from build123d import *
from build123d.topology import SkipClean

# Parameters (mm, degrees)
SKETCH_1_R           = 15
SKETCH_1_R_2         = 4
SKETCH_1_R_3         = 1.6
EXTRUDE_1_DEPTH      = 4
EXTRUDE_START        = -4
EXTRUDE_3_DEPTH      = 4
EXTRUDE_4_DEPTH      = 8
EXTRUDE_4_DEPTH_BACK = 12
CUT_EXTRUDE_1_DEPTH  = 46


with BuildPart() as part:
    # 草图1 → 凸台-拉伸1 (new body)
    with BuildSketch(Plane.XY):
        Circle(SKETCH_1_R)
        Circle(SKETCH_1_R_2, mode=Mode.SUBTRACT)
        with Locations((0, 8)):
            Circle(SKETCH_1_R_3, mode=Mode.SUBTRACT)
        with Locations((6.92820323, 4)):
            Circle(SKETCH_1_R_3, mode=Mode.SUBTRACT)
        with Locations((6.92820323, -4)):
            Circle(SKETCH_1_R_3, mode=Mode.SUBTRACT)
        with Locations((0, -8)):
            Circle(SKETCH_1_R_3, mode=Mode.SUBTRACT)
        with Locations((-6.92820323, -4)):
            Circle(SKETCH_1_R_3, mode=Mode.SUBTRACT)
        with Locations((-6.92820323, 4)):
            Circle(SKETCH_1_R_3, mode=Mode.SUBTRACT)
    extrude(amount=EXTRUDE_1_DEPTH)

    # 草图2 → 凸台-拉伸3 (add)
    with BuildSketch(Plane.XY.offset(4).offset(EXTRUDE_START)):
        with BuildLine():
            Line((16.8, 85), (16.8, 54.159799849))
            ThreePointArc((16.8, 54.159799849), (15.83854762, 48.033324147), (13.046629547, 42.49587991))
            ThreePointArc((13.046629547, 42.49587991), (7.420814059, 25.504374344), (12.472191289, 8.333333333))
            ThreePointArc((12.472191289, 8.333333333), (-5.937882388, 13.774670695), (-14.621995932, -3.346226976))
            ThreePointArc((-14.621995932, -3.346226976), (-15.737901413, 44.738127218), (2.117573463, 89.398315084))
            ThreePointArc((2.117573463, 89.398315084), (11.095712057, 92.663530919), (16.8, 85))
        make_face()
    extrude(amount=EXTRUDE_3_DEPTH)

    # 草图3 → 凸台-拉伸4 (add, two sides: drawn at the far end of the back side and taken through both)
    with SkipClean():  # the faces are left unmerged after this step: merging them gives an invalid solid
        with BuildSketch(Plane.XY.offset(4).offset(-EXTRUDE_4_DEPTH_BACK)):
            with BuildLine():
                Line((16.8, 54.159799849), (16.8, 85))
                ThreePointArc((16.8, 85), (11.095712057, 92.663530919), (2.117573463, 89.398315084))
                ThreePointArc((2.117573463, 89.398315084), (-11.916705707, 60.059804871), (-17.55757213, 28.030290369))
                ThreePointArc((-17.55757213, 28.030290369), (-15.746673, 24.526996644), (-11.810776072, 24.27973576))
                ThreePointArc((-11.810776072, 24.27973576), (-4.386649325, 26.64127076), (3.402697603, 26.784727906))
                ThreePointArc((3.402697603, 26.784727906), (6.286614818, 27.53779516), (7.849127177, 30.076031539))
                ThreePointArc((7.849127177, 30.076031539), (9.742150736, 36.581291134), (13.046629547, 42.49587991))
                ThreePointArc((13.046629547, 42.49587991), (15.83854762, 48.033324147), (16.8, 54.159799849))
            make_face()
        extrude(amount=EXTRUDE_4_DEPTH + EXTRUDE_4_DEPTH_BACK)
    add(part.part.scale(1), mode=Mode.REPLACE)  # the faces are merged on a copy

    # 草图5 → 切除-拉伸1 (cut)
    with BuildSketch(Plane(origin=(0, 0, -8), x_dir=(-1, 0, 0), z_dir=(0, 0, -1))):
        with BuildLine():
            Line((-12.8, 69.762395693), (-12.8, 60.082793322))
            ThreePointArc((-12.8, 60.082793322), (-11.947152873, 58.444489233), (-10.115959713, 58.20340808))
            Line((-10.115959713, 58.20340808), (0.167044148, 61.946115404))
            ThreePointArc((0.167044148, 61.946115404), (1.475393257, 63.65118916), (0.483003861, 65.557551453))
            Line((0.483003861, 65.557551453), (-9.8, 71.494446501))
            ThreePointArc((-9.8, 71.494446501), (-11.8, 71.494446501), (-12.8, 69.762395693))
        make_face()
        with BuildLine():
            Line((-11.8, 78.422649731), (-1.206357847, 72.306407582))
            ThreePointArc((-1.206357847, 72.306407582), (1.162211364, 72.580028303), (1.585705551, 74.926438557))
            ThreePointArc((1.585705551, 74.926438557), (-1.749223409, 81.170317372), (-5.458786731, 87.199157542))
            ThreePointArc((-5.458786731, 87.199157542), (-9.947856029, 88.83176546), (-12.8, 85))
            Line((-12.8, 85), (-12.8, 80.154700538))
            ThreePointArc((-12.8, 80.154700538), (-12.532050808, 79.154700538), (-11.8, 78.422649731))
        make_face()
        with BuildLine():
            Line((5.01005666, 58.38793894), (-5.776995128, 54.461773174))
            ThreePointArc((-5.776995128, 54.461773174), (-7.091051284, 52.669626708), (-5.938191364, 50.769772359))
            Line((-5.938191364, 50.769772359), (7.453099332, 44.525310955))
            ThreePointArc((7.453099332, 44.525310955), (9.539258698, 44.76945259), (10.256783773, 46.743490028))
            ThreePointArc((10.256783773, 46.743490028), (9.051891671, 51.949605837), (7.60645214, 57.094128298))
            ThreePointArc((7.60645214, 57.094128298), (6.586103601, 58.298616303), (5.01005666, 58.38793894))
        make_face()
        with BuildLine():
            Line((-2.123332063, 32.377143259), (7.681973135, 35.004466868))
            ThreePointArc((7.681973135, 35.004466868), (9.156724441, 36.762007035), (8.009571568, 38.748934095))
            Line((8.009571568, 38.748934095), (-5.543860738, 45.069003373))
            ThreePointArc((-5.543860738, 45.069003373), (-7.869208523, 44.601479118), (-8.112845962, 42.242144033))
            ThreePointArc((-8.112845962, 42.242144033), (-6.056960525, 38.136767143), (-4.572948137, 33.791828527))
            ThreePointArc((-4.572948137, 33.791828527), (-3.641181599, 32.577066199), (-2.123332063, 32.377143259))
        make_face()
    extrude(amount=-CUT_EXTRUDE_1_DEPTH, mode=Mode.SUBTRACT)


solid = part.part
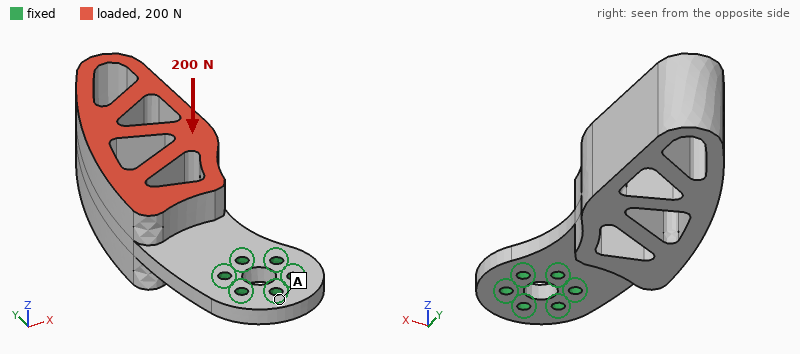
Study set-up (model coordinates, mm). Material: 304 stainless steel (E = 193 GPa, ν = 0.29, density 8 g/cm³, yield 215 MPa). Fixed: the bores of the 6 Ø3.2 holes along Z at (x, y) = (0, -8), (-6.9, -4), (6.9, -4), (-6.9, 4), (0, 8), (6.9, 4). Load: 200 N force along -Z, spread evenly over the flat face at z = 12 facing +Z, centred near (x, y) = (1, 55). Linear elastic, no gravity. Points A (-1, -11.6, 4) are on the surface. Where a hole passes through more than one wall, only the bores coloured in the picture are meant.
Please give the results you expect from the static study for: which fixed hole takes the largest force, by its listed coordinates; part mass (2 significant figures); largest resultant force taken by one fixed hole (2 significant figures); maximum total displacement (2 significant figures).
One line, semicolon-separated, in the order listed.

(0, 8); 210 g; 640 N; 0.42 mm
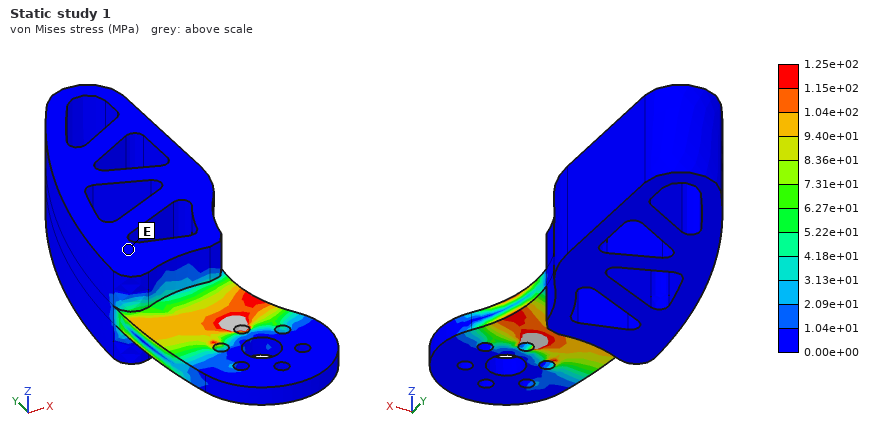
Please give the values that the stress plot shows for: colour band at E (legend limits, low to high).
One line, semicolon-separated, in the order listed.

0.00e+00 to 1.04e+01 MPa
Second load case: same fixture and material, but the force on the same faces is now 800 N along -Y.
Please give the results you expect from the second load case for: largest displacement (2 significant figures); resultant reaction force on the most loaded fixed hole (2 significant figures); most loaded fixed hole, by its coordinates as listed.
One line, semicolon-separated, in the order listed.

0.44 mm; 590 N; (0, 8)
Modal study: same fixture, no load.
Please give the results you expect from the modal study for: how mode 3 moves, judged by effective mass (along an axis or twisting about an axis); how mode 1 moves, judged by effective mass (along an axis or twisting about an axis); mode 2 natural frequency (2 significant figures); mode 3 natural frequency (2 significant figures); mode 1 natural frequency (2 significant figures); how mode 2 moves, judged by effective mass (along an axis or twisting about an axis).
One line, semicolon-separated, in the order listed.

twisting about Y; along Z; 1600 Hz; 1900 Hz; 330 Hz; along X
